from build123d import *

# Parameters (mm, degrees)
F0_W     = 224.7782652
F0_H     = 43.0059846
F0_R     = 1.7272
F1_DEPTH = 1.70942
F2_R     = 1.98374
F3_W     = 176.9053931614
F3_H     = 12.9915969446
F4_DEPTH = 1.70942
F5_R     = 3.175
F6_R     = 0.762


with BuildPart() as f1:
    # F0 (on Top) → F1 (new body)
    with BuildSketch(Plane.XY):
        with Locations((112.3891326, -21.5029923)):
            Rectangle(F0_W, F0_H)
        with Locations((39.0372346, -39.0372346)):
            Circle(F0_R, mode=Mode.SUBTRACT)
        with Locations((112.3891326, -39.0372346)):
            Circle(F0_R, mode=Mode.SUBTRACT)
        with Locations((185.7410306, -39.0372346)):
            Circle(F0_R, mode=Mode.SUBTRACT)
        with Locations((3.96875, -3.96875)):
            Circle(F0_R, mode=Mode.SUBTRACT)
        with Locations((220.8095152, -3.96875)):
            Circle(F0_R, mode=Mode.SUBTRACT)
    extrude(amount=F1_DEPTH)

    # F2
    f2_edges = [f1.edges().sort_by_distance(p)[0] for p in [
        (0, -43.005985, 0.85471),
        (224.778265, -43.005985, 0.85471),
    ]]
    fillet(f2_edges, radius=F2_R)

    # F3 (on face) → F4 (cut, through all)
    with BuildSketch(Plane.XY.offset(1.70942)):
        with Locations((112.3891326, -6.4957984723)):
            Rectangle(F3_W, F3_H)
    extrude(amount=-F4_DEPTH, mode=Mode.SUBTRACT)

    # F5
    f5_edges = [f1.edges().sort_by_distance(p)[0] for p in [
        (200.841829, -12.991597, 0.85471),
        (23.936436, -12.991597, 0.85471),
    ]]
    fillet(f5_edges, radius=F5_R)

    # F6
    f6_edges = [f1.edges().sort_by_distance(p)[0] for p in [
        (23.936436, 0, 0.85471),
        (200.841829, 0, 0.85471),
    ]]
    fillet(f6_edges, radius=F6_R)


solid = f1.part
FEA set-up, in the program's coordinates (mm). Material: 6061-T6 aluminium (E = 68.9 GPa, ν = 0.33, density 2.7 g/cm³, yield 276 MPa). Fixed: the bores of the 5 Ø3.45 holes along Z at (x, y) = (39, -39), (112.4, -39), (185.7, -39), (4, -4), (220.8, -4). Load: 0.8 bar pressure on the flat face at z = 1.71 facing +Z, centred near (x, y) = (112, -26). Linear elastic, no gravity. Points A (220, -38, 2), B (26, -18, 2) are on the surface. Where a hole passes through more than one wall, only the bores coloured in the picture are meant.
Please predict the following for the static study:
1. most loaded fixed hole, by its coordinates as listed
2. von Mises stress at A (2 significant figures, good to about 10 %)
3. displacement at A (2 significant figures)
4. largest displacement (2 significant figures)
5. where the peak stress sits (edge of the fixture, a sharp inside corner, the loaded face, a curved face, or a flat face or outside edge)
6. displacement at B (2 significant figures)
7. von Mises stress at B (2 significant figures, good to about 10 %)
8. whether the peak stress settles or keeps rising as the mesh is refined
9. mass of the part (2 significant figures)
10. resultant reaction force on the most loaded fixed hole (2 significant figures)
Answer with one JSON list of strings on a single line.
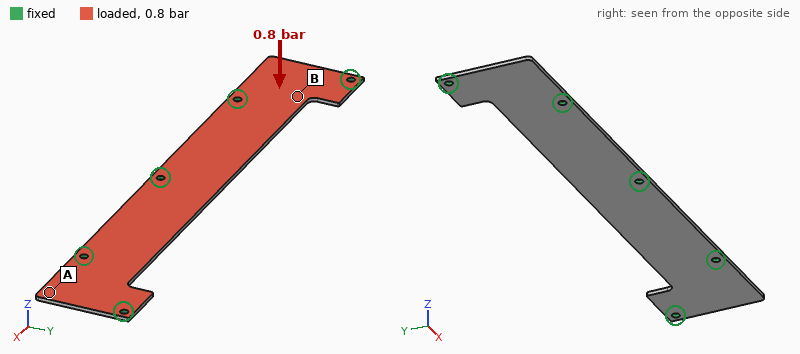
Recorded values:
["(112.4, -39)", "12 MPa", "0.12 mm", "0.51 mm", "edge of the fixture", "0.086 mm", "38 MPa", "keeps rising", "34 g", "180 N"]
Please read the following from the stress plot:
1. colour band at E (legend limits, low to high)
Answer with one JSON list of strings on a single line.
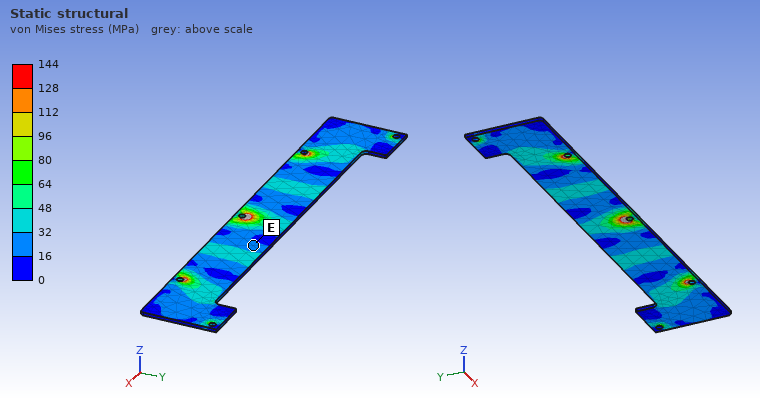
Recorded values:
["16 to 32 MPa"]
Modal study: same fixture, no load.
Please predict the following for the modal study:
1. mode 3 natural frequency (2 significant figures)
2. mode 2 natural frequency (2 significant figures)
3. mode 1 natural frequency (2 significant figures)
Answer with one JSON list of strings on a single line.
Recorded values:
["1800 Hz", "1200 Hz", "1200 Hz"]
